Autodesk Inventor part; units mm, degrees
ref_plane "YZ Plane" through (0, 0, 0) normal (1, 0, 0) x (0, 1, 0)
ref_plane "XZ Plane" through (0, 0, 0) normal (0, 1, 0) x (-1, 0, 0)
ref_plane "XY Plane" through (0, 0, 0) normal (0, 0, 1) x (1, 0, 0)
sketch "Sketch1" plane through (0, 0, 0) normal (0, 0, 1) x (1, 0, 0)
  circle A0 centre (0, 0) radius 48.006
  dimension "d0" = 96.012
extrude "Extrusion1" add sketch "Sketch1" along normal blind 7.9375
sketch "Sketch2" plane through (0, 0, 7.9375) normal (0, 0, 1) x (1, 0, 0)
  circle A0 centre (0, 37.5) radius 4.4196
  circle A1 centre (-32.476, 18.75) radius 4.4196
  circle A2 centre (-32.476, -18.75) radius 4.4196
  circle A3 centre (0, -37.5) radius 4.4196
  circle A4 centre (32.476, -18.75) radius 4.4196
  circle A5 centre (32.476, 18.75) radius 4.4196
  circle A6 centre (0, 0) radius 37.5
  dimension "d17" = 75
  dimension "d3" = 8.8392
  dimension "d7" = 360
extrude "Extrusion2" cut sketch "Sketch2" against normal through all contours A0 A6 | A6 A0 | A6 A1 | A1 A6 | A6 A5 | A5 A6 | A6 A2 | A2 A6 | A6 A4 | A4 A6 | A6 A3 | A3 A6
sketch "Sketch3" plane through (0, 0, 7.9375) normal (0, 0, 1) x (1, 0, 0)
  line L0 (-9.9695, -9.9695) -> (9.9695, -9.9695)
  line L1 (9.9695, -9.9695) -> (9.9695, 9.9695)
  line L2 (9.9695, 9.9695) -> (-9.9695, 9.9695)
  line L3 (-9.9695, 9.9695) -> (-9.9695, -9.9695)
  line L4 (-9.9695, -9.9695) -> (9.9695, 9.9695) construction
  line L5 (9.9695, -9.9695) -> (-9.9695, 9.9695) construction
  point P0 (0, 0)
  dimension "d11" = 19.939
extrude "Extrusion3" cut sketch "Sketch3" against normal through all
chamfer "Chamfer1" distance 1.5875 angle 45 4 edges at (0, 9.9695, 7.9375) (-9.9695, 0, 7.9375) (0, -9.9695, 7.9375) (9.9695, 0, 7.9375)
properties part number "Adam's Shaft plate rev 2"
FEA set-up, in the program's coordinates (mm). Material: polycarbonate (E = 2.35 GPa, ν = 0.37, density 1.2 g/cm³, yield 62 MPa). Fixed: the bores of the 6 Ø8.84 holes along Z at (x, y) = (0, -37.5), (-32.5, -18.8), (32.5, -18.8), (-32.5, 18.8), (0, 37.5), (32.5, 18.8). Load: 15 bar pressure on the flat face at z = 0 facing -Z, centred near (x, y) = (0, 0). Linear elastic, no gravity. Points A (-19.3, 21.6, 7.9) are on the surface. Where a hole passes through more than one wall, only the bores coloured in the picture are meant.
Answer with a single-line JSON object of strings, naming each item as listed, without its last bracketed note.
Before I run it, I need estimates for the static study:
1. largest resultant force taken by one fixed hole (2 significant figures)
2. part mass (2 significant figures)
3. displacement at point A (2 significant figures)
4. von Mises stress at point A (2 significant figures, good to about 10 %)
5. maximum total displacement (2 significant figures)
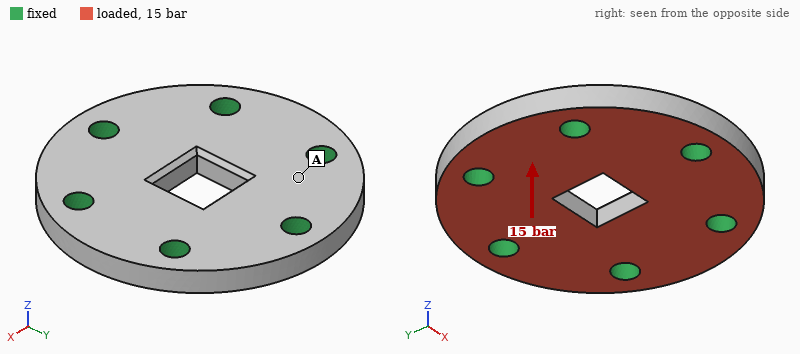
{"largest resultant force taken by one fixed hole": "1.6 kN", "part mass": "62 g", "displacement at point A": "0.13 mm", "von Mises stress at point A": "9.4 MPa", "maximum total displacement": "0.43 mm"}
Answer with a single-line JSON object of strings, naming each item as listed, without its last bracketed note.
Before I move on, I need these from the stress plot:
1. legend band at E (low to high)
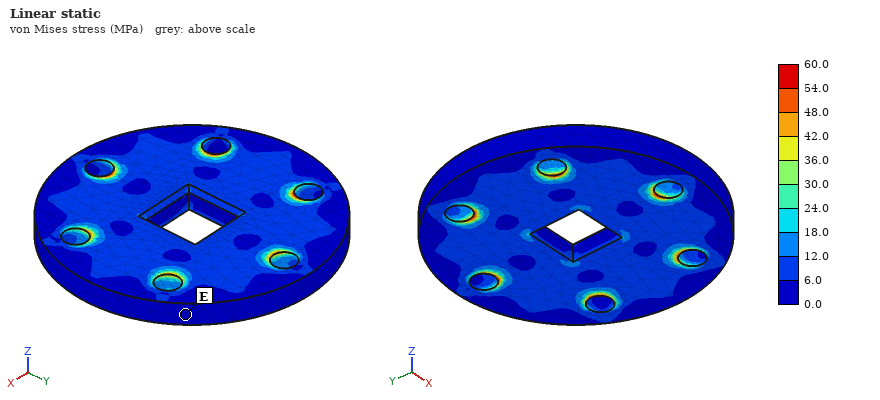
{"legend band at E": "0.0 to 6.0 MPa"}
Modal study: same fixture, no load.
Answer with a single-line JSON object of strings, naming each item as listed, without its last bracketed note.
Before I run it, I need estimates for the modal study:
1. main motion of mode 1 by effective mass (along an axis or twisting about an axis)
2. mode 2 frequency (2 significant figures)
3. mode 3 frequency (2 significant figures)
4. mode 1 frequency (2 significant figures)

{"main motion of mode 1 by effective mass": "along Z", "mode 2 frequency": "5700 Hz", "mode 3 frequency": "5700 Hz", "mode 1 frequency": "3800 Hz"}
